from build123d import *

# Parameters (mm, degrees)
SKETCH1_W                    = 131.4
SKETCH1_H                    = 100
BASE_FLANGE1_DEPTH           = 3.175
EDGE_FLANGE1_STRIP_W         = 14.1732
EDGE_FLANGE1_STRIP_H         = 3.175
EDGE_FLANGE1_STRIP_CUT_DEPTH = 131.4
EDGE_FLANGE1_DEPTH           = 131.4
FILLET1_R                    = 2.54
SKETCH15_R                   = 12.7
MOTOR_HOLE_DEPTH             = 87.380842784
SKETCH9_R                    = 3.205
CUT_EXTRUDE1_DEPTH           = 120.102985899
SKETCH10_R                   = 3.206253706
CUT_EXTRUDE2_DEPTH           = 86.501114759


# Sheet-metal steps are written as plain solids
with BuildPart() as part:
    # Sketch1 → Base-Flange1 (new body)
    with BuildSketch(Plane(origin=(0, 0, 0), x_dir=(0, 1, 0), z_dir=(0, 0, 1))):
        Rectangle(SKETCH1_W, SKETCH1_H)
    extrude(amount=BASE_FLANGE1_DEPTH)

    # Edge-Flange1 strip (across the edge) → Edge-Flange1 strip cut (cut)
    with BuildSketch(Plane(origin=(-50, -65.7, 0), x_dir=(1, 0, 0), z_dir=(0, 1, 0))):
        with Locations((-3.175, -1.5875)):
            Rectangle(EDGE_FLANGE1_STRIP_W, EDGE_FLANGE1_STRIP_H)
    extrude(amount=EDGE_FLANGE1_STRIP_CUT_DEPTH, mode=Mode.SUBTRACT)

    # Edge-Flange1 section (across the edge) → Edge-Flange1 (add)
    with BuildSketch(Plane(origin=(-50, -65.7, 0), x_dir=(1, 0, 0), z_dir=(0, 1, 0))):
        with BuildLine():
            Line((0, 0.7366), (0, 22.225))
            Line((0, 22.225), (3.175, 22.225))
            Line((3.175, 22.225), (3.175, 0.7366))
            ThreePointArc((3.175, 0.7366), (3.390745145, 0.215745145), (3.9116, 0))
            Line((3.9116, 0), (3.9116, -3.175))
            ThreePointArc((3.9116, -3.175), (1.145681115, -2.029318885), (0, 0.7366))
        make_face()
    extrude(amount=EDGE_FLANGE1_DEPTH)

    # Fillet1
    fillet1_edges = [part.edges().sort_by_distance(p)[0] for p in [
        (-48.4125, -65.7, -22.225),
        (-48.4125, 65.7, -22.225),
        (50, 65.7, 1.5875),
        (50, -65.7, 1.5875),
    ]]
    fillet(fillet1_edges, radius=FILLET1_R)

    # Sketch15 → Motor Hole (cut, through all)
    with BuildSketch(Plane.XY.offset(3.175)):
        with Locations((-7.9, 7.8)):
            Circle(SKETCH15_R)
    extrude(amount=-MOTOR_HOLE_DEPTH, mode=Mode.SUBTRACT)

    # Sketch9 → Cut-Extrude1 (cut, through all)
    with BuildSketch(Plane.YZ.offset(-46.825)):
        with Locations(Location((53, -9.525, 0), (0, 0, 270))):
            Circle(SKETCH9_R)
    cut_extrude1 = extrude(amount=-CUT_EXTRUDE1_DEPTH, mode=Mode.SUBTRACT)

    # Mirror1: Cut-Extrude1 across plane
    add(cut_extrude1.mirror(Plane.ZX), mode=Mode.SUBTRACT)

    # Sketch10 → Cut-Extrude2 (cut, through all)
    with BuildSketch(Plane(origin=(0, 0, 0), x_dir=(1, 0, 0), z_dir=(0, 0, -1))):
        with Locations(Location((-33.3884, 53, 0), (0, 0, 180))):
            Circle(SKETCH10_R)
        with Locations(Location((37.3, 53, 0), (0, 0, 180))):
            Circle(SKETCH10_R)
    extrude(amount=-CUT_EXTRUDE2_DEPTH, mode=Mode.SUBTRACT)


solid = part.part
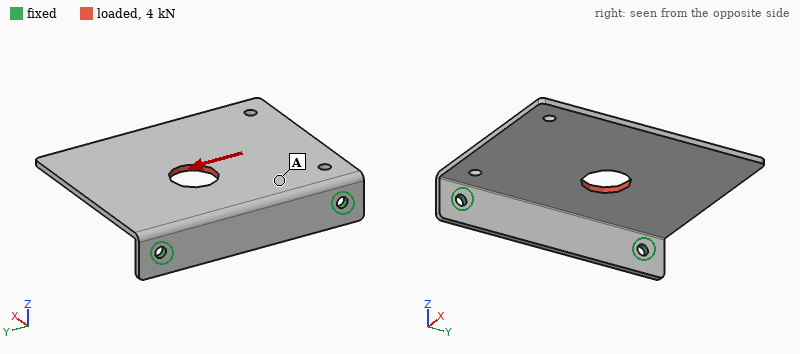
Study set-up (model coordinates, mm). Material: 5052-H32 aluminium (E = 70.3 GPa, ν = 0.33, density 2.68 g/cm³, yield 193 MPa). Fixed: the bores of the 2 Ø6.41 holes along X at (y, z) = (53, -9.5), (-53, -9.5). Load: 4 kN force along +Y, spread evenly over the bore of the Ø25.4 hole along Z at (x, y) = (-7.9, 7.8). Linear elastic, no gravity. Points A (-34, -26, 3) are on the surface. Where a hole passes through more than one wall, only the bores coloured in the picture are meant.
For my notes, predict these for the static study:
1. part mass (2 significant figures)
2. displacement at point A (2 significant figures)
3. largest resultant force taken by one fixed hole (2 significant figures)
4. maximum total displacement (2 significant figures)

130 g
0.074 mm
2.6 kN
0.46 mm
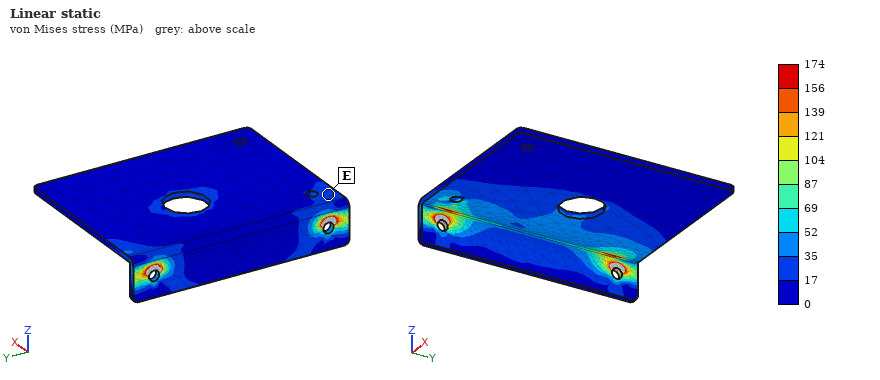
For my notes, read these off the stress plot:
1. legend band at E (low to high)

17 to 35 MPa
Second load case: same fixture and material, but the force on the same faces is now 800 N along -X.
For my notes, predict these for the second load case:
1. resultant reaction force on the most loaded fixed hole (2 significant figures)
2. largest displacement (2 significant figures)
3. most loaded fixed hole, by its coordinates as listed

470 N
0.31 mm
(53, -9.5)
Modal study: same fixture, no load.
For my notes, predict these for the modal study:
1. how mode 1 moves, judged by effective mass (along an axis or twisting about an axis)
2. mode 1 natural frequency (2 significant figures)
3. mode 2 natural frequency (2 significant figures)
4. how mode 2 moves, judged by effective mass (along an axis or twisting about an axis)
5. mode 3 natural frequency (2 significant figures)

along Z
210 Hz
490 Hz
twisting about X
1300 Hz
